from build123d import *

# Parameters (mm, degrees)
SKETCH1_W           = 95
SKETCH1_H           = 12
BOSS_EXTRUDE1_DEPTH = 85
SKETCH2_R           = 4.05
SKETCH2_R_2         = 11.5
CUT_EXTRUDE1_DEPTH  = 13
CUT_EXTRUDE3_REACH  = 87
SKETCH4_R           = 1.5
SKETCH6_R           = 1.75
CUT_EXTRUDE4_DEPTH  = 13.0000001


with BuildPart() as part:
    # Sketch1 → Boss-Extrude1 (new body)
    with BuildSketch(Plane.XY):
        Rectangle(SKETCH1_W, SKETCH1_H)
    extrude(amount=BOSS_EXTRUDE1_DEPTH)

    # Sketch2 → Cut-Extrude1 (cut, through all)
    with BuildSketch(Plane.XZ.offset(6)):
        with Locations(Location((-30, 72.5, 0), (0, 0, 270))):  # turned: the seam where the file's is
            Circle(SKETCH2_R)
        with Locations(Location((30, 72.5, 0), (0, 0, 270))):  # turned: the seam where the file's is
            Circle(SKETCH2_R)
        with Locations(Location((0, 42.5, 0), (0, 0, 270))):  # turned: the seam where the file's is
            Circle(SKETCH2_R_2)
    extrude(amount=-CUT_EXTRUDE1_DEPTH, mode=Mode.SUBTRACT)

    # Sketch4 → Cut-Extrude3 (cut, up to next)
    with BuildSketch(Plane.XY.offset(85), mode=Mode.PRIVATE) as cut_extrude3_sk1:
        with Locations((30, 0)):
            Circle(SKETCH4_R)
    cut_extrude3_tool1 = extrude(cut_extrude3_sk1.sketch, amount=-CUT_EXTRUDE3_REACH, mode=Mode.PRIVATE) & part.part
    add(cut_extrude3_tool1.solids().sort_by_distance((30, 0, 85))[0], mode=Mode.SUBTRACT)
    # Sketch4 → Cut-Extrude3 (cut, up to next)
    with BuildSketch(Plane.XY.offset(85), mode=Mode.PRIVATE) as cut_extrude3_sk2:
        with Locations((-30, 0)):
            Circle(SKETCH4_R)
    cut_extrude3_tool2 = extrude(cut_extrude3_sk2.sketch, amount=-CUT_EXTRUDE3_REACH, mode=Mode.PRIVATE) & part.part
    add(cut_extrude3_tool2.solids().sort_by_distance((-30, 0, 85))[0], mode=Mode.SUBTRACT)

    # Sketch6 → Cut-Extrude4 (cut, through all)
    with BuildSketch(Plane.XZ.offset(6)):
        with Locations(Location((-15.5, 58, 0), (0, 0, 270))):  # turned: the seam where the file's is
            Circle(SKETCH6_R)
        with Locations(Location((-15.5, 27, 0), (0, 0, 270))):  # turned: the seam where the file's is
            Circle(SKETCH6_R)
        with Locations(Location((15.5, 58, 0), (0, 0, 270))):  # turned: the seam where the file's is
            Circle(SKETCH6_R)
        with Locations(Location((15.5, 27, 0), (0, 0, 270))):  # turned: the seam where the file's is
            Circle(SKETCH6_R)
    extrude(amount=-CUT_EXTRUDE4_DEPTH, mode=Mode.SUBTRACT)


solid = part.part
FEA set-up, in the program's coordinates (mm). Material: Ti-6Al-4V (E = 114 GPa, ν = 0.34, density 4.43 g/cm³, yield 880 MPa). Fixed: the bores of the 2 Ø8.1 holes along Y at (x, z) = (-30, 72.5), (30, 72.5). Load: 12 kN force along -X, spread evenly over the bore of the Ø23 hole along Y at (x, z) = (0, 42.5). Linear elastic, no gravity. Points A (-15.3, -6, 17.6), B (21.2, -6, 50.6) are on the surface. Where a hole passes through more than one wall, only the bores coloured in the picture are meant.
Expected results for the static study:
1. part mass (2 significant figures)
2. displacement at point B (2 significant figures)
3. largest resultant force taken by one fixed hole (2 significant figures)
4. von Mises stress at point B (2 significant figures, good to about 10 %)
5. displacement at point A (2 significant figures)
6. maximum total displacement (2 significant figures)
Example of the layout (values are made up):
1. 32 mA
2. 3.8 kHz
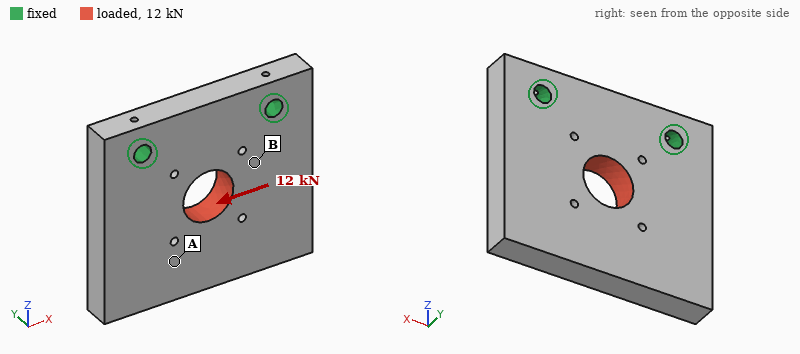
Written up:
1. 400 g
2. 9.3 µm
3. 8.0 kN
4. 23 MPa
5. 19 µm
6. 23 µm
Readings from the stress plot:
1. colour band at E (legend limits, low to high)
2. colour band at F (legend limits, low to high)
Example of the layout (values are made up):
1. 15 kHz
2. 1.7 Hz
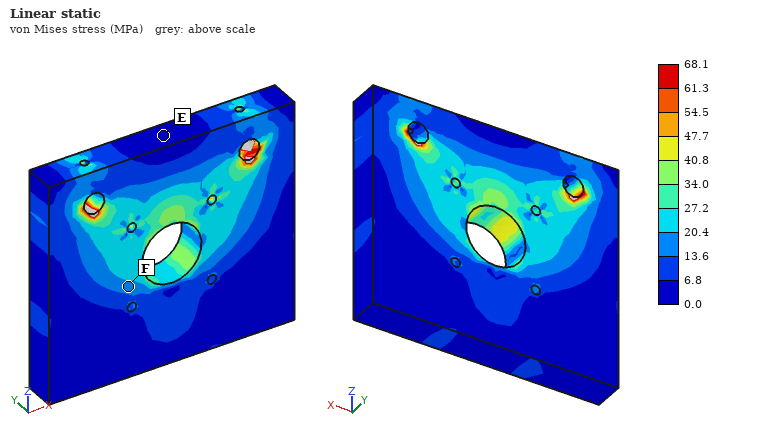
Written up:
1. 0.0 to 6.8 MPa
2. 13.6 to 20.4 MPa
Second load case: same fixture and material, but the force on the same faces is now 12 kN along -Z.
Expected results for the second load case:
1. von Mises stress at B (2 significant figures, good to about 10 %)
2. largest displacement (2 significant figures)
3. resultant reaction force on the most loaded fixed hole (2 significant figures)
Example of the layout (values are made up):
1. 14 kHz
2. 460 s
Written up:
1. 16 MPa
2. 8.6 µm
3. 6.2 kN
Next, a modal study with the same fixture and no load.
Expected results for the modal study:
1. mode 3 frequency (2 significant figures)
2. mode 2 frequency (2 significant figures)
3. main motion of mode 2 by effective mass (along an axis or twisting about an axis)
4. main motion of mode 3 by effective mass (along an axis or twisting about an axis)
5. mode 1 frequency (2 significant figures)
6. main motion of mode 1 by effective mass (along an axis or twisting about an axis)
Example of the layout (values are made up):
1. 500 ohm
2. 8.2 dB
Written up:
1. 6300 Hz
2. 3300 Hz
3. twisting about Z
4. along X
5. 1600 Hz
6. along Y
